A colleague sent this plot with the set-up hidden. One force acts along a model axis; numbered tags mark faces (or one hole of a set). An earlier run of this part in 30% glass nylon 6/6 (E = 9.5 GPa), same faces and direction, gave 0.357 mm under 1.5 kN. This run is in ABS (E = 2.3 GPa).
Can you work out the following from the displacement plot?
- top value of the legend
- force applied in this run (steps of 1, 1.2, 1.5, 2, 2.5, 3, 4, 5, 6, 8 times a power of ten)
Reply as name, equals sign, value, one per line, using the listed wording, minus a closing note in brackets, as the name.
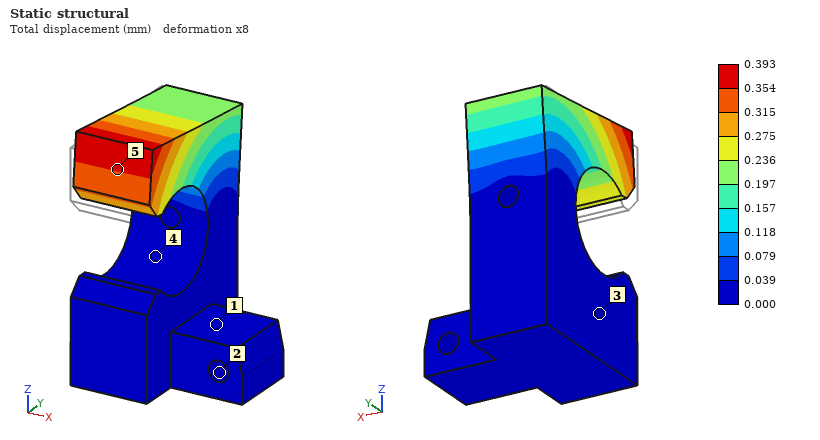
top value of the legend = 0.393 mm
force applied in this run = 400 N
